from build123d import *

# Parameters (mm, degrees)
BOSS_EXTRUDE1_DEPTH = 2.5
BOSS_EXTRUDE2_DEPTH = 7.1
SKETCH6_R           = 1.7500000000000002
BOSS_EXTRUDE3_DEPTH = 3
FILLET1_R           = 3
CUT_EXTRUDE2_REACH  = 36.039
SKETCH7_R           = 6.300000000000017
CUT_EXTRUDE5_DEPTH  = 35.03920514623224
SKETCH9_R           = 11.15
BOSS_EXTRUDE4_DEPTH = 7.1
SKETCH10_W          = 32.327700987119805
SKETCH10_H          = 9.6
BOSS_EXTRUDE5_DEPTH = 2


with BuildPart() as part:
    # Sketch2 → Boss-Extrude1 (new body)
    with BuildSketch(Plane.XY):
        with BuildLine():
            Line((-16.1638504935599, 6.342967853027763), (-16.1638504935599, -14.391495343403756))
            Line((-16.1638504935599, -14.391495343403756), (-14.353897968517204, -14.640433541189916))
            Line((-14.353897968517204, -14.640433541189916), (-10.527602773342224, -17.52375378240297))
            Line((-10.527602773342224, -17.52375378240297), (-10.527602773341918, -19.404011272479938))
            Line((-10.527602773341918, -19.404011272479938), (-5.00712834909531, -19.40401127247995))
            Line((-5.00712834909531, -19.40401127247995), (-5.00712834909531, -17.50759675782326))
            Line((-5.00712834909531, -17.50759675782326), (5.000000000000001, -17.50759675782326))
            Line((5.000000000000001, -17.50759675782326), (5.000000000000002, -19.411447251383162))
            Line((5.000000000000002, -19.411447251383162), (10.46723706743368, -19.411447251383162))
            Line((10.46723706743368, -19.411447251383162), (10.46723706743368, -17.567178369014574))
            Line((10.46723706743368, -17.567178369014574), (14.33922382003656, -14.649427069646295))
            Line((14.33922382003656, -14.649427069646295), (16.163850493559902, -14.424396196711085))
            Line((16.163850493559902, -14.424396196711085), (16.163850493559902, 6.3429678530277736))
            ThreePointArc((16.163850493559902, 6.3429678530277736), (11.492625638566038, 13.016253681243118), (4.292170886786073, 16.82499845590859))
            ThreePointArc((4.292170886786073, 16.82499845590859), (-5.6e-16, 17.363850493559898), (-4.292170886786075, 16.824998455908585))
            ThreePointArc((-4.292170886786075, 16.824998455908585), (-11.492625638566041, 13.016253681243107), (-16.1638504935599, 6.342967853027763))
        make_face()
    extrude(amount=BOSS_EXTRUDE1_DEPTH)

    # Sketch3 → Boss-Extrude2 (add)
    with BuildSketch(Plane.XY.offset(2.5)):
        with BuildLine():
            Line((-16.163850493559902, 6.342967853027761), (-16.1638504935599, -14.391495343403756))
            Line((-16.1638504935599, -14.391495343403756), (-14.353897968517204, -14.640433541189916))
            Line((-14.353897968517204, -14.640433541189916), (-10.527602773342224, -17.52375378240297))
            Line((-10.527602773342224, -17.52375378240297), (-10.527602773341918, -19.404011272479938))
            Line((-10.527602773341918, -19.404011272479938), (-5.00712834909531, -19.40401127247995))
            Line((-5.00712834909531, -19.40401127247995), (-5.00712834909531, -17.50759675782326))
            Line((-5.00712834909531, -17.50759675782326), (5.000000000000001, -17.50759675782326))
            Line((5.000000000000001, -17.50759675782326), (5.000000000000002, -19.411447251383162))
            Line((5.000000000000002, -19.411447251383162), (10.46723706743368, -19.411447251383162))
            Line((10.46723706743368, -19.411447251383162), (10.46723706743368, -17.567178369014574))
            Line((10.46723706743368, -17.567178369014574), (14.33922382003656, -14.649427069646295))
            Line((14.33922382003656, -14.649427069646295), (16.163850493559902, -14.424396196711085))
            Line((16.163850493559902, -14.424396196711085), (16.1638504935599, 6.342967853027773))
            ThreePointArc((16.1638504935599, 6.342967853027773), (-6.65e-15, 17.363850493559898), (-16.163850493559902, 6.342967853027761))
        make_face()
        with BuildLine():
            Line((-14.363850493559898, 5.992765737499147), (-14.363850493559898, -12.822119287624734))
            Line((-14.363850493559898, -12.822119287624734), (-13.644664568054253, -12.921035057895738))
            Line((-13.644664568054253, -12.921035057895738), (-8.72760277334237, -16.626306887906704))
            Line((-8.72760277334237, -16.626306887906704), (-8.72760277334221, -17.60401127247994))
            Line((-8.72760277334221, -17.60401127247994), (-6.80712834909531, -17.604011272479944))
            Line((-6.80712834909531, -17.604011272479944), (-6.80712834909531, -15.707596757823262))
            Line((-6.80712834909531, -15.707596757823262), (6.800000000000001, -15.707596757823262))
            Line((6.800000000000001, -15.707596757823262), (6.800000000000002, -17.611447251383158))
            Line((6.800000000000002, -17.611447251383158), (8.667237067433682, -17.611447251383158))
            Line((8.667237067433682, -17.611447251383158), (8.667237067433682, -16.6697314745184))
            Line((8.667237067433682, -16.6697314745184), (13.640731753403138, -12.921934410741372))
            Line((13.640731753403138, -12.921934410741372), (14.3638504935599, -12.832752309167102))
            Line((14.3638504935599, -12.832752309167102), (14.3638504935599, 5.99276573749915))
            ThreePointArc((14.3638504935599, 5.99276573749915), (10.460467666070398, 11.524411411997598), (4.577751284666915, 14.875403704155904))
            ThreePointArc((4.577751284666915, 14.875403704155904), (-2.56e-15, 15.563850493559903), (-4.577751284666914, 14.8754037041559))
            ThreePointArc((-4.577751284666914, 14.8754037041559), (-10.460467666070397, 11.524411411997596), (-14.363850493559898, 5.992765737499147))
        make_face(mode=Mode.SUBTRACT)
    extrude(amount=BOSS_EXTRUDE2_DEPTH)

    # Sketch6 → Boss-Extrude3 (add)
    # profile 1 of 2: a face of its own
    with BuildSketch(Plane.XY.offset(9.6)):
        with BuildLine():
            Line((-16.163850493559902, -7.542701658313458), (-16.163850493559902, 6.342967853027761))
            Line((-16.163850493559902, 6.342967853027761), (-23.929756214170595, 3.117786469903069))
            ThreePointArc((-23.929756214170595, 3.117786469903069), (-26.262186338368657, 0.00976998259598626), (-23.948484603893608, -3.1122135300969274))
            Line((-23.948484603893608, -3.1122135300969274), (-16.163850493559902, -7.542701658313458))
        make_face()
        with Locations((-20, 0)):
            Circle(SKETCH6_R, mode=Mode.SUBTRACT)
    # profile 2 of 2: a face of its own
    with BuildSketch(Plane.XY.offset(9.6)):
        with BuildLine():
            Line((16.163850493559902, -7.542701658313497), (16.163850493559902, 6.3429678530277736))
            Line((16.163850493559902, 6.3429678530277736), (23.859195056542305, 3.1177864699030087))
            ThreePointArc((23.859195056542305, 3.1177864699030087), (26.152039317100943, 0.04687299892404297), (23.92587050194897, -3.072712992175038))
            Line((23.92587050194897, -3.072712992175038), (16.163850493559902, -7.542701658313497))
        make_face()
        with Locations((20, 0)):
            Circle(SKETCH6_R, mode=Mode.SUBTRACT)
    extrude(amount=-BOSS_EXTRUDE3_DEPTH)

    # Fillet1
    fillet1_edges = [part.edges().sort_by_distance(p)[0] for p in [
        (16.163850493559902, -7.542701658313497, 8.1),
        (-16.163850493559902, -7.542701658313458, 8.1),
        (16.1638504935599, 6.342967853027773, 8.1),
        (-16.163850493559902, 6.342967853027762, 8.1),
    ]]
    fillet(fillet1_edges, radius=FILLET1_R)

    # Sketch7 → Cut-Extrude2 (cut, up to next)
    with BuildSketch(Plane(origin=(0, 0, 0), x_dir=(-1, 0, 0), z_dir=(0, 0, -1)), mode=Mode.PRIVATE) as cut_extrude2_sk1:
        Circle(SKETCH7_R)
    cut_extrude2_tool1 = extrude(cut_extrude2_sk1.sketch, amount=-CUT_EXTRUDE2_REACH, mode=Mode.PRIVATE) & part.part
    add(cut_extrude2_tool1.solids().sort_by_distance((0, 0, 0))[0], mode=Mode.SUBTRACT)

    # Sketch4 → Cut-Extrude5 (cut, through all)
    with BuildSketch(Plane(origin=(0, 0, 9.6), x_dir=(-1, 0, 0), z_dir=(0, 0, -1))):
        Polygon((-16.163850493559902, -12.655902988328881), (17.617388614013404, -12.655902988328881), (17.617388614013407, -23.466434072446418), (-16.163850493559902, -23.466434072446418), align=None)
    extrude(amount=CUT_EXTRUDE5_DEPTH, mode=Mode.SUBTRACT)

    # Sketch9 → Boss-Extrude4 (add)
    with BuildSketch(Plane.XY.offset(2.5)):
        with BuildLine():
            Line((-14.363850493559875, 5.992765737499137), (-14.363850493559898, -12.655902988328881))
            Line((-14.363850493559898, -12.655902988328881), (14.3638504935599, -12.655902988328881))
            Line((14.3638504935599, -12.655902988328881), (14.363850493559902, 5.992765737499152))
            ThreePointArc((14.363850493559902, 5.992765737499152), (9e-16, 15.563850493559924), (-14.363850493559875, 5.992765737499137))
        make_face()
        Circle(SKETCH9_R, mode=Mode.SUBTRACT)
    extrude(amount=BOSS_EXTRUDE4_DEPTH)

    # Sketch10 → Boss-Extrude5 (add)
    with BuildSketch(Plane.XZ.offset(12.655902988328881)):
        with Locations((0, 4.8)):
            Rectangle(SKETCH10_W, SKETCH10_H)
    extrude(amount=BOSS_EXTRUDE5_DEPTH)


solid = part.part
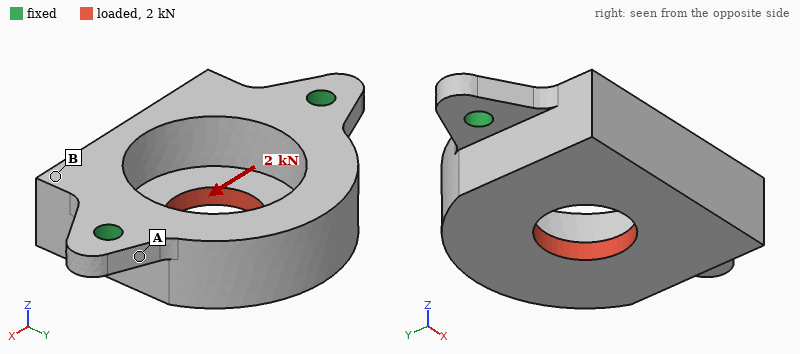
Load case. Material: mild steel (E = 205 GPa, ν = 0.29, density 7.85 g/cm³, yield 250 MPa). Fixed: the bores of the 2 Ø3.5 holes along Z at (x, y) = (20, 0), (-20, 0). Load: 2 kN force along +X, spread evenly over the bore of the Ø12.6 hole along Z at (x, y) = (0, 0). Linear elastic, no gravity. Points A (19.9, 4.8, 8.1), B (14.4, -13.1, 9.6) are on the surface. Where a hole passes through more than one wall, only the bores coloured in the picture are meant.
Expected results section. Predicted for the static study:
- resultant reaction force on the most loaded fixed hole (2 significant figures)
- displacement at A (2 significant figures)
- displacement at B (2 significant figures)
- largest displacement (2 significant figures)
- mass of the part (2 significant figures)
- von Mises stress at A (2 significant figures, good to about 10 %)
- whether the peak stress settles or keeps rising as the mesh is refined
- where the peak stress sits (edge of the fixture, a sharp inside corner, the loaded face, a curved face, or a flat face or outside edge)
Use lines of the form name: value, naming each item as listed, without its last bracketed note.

resultant reaction force on the most loaded fixed hole: 1.1 kN
displacement at A: 0.70 µm
displacement at B: 1.9 µm
largest displacement: 4.2 µm
mass of the part: 50 g
von Mises stress at A: 26 MPa
whether the peak stress settles or keeps rising as the mesh is refined: keeps rising
where the peak stress sits: edge of the fixture
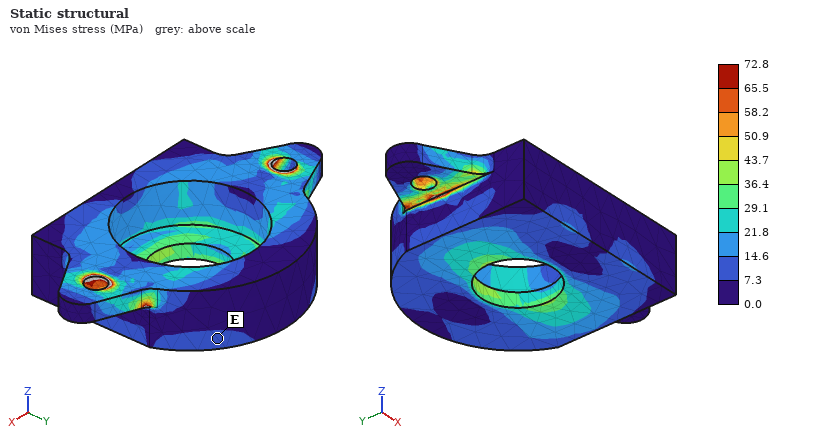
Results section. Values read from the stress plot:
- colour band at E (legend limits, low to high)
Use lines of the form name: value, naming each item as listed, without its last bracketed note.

colour band at E: 7.3 to 14.6 MPa
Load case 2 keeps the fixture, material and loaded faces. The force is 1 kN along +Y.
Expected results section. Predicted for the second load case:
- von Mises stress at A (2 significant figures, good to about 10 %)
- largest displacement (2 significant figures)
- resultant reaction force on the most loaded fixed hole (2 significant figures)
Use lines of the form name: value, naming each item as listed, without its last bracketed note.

von Mises stress at A: 73 MPa
largest displacement: 30 µm
resultant reaction force on the most loaded fixed hole: 500 N
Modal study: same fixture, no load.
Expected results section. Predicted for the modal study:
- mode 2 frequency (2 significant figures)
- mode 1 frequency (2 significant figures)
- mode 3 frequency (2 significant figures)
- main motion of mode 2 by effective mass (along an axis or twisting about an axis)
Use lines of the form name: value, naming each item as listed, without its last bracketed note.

mode 2 frequency: 12 kHz
mode 1 frequency: 4600 Hz
mode 3 frequency: 19 kHz
main motion of mode 2 by effective mass: along Z
